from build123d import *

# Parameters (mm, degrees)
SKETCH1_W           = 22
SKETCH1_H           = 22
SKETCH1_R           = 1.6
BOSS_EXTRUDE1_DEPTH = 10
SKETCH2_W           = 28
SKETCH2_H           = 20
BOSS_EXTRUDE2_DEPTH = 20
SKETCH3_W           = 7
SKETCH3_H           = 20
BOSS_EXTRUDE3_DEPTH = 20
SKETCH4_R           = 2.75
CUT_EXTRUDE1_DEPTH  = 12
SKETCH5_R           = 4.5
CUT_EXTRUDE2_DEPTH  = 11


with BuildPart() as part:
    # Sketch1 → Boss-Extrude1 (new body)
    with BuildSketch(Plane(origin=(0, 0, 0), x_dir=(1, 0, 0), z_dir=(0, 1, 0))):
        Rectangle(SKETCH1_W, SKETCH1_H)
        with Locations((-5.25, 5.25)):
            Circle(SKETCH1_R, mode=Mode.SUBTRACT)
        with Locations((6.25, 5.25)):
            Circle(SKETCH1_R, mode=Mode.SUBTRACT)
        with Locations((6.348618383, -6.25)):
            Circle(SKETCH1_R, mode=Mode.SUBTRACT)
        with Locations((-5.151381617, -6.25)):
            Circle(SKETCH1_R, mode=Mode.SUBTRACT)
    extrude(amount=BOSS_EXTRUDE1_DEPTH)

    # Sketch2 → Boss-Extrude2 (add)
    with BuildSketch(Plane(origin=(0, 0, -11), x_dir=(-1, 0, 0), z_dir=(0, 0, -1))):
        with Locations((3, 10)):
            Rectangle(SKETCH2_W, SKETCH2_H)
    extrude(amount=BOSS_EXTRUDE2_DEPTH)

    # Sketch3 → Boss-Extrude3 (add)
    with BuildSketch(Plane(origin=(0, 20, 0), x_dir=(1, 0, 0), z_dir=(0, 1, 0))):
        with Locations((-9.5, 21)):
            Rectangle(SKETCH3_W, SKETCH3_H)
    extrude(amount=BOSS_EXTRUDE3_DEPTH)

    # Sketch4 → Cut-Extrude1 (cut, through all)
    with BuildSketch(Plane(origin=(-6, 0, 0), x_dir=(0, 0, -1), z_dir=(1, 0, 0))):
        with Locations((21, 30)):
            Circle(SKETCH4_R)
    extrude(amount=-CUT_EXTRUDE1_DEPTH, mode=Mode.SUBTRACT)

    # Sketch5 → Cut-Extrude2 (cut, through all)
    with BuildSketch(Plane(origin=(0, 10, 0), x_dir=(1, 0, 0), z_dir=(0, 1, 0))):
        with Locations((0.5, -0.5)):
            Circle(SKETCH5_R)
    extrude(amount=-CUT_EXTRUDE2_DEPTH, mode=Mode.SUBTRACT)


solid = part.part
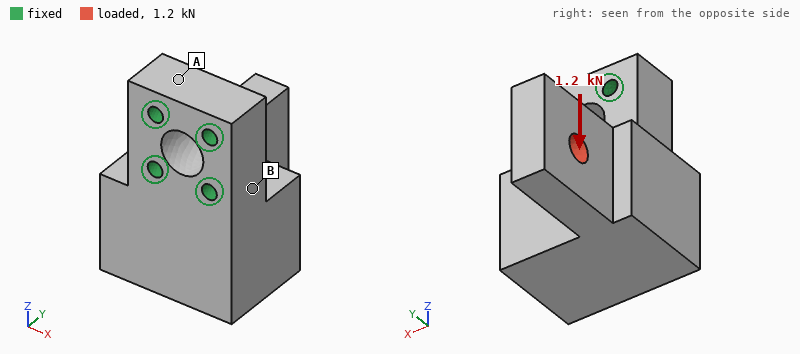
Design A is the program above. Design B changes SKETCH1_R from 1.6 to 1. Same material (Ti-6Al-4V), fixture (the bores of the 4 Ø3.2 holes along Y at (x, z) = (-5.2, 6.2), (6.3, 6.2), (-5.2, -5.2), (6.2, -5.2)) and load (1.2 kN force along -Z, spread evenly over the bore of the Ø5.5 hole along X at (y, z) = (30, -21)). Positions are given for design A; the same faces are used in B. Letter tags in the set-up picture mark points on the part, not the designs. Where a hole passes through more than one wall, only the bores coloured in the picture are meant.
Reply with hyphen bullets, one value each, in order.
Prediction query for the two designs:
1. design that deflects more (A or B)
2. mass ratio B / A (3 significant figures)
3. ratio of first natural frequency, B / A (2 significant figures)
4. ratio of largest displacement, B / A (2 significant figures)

- B
- 1.01
- 0.93
- 1.1
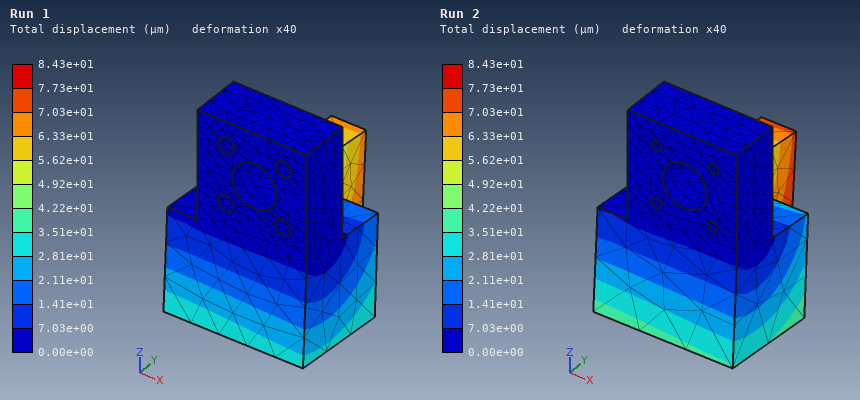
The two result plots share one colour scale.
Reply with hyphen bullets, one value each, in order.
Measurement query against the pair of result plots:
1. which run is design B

- Run 2
